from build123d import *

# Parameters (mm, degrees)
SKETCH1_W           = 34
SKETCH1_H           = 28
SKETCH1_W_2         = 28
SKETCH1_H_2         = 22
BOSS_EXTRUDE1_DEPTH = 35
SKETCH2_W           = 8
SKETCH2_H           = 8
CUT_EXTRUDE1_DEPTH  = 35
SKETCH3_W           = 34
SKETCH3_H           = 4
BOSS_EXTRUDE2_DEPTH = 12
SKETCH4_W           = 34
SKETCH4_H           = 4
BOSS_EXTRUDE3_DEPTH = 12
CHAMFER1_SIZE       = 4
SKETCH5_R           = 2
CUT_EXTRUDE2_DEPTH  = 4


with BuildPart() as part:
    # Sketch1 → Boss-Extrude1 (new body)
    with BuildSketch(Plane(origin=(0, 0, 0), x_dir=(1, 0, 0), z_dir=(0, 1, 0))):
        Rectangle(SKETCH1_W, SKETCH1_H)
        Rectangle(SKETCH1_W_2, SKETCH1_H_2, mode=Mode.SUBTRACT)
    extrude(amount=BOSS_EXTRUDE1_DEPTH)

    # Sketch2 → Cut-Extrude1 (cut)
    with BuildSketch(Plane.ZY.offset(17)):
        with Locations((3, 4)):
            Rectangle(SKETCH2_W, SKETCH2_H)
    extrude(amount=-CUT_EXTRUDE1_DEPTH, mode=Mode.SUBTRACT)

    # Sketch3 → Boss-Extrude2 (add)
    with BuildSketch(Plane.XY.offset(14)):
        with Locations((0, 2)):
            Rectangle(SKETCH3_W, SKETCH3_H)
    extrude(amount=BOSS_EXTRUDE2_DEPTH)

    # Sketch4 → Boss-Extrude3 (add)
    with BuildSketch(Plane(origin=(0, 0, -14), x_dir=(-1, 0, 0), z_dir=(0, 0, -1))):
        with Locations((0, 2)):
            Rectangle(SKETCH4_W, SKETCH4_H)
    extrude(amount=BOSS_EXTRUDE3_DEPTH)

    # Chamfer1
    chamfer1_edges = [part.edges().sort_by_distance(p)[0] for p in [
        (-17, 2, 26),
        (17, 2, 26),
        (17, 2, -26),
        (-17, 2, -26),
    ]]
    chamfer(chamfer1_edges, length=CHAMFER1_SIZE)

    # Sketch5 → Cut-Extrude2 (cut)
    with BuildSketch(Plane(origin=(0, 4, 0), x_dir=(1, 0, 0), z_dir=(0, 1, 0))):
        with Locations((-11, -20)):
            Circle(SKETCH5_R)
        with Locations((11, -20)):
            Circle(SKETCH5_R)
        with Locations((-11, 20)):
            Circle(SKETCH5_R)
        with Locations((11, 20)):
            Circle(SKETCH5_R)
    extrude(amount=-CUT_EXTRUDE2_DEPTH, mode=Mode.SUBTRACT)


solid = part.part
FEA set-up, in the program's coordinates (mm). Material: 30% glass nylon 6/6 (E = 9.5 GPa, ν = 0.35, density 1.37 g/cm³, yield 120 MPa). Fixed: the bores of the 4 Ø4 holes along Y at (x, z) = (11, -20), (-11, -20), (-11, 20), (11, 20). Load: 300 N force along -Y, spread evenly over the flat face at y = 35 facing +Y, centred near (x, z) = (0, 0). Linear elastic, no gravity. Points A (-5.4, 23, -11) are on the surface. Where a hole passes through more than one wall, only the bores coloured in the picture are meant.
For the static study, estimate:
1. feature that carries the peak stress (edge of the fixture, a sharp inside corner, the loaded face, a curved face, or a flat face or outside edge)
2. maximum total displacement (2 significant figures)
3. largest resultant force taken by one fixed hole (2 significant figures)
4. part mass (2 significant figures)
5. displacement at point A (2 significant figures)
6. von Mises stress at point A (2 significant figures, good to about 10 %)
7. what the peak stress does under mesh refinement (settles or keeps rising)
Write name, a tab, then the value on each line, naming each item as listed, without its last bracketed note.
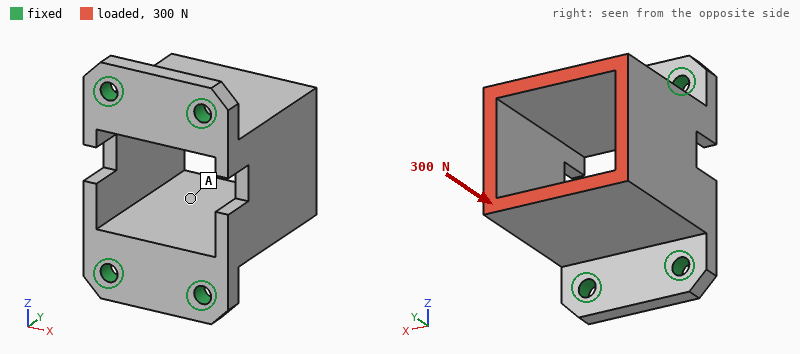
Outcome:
feature that carries the peak stress	edge of the fixture
maximum total displacement	13 µm
largest resultant force taken by one fixed hole	79 N
part mass	20 g
displacement at point A	11 µm
von Mises stress at point A	1.3 MPa
what the peak stress does under mesh refinement	keeps rising
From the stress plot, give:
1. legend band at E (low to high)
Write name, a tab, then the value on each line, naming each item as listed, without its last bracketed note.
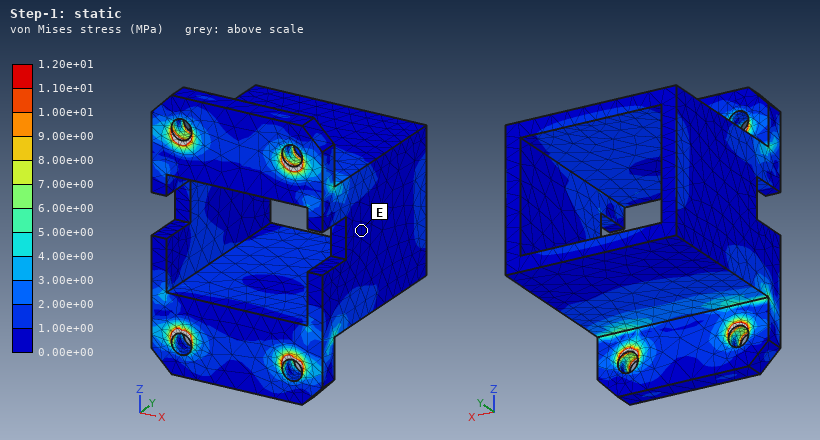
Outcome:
legend band at E	0.00e+00 to 1.00e+00 MPa
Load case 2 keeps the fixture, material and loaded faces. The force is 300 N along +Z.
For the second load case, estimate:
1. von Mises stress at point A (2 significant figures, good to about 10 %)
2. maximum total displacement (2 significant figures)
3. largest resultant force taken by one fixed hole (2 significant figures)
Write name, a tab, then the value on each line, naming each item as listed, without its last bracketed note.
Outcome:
von Mises stress at point A	4.3 MPa
maximum total displacement	0.13 mm
largest resultant force taken by one fixed hole	180 N
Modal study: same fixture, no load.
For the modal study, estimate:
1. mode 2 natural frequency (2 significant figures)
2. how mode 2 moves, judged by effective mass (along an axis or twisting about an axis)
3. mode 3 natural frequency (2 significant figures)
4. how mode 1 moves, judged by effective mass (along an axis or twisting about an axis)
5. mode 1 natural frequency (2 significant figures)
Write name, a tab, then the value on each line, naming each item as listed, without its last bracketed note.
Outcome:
mode 2 natural frequency	4300 Hz
how mode 2 moves, judged by effective mass	along Z
mode 3 natural frequency	4700 Hz
how mode 1 moves, judged by effective mass	along X
mode 1 natural frequency	3400 Hz
